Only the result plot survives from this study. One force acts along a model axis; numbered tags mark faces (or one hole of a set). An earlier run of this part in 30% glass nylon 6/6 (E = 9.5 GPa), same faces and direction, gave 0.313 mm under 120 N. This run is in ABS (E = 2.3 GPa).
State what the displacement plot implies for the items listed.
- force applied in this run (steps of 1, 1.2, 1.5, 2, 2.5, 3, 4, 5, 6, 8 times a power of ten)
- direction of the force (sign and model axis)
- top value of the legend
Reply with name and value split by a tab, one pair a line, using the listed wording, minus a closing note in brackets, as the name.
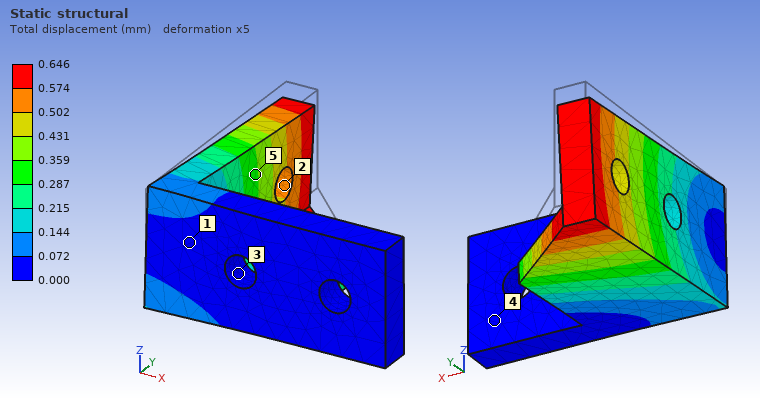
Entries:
force applied in this run	60 N
direction of the force	-Z
top value of the legend	0.646 mm
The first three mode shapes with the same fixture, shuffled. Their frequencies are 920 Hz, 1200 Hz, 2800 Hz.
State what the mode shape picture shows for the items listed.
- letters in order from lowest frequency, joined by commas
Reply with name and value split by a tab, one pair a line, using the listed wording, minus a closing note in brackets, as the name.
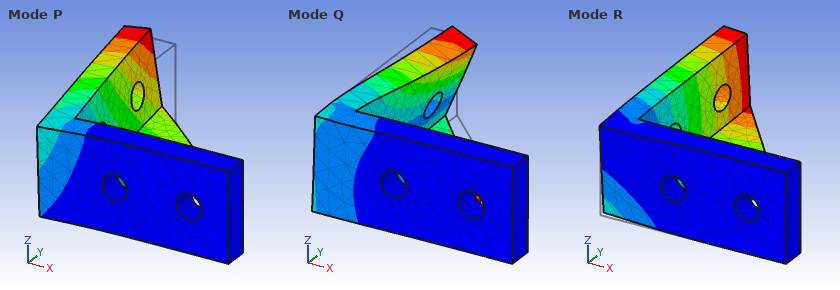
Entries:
letters in order from lowest frequency, joined by commas	R, P, Q
